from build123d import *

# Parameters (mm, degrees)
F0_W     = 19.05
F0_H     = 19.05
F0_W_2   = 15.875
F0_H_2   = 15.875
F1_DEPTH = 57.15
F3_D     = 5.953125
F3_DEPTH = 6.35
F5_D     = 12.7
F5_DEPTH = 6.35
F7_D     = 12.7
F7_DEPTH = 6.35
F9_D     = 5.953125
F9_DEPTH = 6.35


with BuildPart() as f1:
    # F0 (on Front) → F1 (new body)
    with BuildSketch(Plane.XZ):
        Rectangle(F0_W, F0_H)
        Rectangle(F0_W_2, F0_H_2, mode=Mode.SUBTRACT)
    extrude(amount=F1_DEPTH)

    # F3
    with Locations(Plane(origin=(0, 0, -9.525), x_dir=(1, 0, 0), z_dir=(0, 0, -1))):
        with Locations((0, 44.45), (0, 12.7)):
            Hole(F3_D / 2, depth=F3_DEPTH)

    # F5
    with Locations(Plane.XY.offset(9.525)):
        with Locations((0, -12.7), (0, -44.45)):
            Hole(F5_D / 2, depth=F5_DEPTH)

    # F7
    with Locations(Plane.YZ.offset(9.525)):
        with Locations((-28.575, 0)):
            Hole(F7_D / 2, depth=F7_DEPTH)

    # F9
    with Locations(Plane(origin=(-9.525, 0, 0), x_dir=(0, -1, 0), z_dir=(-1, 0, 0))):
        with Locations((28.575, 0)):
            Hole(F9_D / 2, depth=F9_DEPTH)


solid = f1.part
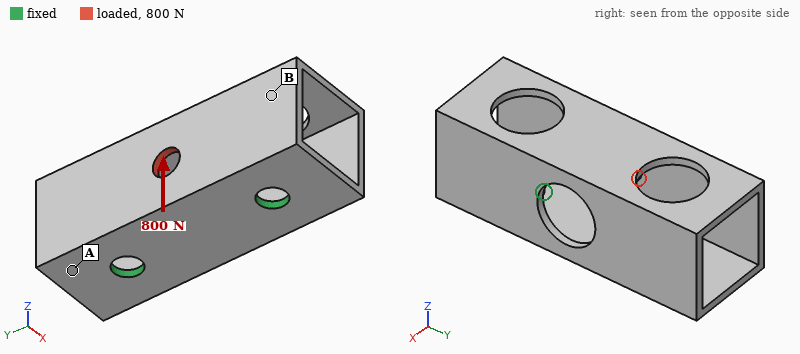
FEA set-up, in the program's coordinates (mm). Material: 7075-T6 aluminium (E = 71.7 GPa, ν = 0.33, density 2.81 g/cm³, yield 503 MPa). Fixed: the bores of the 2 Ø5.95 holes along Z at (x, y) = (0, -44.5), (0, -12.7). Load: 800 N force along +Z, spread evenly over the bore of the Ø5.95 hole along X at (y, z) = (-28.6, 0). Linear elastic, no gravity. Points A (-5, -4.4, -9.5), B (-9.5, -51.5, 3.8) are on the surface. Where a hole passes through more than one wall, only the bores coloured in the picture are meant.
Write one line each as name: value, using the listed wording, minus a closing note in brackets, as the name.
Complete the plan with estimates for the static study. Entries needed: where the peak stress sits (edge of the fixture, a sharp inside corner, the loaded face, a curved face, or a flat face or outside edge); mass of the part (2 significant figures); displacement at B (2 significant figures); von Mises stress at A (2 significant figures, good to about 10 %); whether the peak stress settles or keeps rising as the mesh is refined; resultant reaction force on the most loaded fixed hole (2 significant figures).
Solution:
where the peak stress sits: edge of the fixture
mass of the part: 16 g
displacement at B: 0.13 mm
von Mises stress at A: 62 MPa
whether the peak stress settles or keeps rising as the mesh is refined: keeps rising
resultant reaction force on the most loaded fixed hole: 430 N
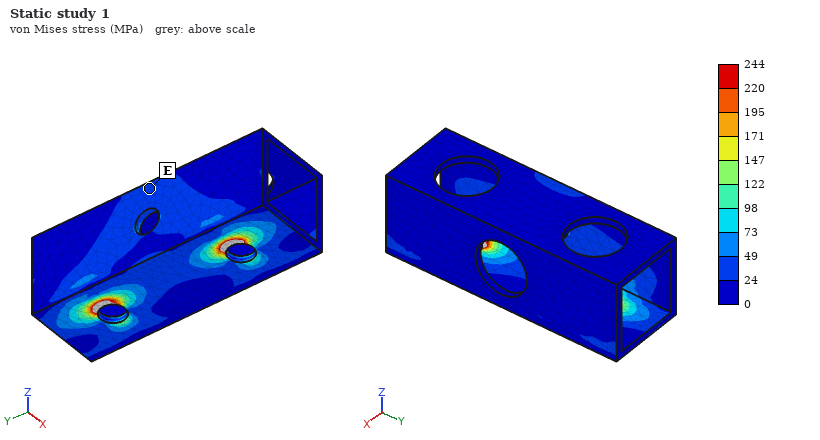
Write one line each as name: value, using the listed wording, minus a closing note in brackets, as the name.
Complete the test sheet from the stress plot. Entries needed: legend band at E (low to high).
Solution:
legend band at E: 24 to 49 MPa
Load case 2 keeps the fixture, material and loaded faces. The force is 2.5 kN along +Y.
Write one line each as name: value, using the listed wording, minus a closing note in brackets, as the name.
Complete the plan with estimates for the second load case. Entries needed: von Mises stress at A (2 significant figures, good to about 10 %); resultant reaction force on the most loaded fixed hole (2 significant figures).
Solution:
von Mises stress at A: 49 MPa
resultant reaction force on the most loaded fixed hole: 1.5 kN
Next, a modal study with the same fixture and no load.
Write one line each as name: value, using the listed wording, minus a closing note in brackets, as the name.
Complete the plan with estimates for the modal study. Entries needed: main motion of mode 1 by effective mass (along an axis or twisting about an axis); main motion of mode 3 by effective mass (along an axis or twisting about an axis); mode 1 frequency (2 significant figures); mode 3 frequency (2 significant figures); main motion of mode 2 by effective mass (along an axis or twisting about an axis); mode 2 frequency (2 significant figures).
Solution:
main motion of mode 1 by effective mass: along X
main motion of mode 3 by effective mass: twisting about Z
mode 1 frequency: 2300 Hz
mode 3 frequency: 6700 Hz
main motion of mode 2 by effective mass: along Y
mode 2 frequency: 5800 Hz
